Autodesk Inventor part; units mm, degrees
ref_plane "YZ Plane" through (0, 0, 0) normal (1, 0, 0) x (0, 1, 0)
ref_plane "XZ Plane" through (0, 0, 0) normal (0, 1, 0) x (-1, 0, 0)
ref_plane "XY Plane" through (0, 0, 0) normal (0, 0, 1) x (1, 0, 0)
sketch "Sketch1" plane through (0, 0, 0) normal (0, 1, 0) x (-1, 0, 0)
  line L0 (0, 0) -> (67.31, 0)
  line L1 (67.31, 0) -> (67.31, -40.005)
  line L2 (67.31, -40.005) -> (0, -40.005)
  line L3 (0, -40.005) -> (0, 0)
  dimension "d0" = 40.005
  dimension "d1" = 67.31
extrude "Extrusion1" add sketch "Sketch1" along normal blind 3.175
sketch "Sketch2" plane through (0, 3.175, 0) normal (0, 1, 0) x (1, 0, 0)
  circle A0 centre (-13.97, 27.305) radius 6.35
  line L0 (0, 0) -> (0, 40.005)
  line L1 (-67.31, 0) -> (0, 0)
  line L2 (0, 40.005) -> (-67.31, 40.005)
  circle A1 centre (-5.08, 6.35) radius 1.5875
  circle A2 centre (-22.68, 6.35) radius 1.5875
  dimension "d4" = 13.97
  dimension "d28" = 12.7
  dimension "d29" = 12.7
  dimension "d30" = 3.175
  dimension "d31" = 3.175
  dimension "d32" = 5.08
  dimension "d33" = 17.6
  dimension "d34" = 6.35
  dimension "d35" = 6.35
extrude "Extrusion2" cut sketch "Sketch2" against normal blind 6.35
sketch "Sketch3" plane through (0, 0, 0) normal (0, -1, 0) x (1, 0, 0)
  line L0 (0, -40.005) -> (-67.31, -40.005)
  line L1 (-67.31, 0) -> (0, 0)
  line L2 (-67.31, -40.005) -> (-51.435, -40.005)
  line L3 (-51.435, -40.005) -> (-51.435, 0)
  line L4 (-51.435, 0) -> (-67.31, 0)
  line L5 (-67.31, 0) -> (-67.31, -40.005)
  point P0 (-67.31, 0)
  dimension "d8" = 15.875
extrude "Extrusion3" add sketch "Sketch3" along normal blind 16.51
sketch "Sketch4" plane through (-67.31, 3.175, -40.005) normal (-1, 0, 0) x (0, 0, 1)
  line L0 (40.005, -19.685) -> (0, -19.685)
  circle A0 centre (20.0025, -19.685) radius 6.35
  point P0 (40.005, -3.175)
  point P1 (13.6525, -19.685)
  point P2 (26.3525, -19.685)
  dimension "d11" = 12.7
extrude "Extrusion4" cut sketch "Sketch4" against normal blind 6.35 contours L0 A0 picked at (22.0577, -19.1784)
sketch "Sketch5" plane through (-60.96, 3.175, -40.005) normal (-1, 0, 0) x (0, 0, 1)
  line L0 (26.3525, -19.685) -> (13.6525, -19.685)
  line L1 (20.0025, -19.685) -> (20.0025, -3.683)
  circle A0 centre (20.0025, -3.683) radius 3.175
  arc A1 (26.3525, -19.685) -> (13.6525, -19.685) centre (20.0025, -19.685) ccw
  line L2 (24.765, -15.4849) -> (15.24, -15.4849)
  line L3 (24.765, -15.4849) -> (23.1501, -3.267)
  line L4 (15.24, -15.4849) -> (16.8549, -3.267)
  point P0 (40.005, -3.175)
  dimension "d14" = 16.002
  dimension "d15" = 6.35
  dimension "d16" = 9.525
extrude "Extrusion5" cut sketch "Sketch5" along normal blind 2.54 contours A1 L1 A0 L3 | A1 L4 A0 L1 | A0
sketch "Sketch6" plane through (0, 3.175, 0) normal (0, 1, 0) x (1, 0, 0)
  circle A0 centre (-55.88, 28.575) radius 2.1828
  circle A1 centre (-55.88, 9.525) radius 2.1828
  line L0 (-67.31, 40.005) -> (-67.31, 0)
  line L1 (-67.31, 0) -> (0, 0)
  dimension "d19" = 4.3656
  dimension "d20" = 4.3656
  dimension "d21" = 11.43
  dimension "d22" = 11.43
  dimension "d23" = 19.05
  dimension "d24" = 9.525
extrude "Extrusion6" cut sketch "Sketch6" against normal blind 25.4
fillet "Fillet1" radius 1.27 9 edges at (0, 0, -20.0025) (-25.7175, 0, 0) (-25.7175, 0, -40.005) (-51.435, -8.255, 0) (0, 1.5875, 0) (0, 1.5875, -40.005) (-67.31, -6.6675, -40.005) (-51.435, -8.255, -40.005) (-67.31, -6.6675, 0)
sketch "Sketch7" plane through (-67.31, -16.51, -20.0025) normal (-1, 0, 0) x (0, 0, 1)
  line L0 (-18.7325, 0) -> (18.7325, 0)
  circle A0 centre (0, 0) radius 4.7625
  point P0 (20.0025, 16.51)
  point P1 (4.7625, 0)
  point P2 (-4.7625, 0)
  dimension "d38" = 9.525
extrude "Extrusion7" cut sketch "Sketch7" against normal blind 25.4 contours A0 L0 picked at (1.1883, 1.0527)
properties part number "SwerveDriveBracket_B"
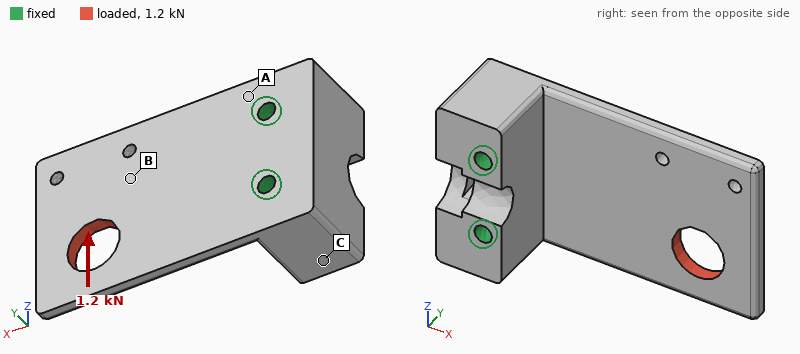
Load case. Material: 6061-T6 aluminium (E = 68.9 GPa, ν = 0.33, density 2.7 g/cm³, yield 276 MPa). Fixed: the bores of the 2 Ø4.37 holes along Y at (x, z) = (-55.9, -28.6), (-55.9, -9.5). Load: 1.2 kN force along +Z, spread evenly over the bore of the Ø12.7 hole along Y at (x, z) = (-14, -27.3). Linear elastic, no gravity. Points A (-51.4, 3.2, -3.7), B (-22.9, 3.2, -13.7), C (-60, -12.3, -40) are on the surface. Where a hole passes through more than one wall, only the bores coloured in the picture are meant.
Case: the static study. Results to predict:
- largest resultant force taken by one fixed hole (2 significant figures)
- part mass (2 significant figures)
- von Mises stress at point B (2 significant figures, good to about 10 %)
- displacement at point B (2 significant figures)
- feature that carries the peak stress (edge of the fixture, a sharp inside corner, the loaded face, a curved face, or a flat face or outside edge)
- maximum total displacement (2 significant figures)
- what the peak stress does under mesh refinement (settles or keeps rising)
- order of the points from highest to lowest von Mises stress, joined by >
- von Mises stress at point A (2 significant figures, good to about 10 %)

2.2 kN
46 g
18 MPa
35 µm
edge of the fixture
73 µm
keeps rising
A > B > C
35 MPa
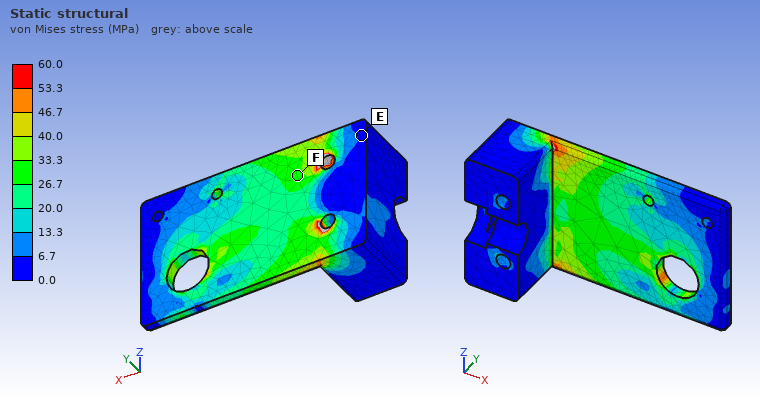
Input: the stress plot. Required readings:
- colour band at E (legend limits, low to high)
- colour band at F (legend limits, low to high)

0.0 to 6.7 MPa
26.7 to 33.3 MPa
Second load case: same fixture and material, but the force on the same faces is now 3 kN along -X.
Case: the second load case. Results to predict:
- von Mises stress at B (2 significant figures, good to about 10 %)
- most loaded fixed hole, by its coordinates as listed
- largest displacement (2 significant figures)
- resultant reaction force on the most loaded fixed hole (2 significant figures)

22 MPa
(-55.9, -28.6)
49 µm
2.6 kN
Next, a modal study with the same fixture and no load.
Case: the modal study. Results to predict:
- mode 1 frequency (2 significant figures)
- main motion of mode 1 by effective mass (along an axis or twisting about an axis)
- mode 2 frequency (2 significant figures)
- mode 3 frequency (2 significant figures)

1000 Hz
along Y
2800 Hz
5500 Hz
